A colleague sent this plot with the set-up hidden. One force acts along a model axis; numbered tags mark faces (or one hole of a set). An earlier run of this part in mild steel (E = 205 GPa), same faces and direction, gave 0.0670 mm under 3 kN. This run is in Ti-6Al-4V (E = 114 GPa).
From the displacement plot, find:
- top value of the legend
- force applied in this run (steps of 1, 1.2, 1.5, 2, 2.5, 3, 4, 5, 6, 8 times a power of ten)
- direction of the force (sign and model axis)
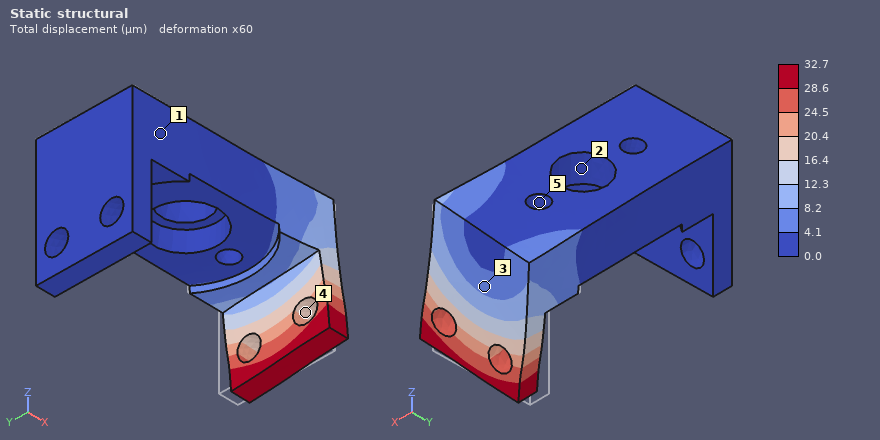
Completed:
32.7 µm
800 N
-Y
